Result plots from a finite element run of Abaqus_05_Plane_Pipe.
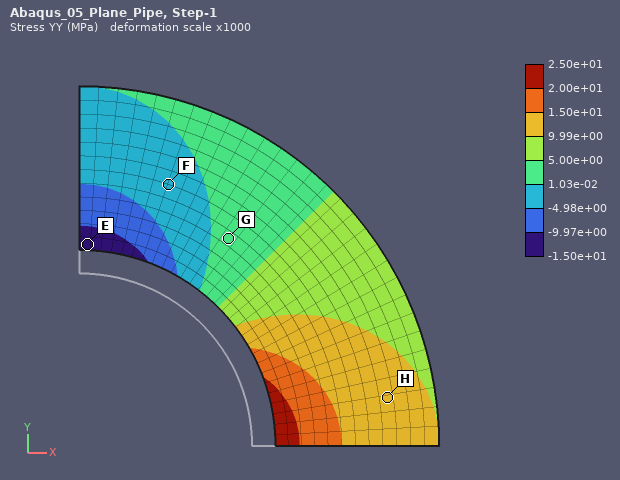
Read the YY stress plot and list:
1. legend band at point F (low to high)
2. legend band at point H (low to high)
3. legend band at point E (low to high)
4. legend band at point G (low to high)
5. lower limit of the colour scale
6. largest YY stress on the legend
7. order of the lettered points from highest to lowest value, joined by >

-4.98e+00 to 1.03e-02 MPa
9.99e+00 to 1.50e+01 MPa
-1.50e+01 to -9.97e+00 MPa
1.03e-02 to 5.00e+00 MPa
-1.50e+01 MPa
2.50e+01 MPa
H > G > F > E
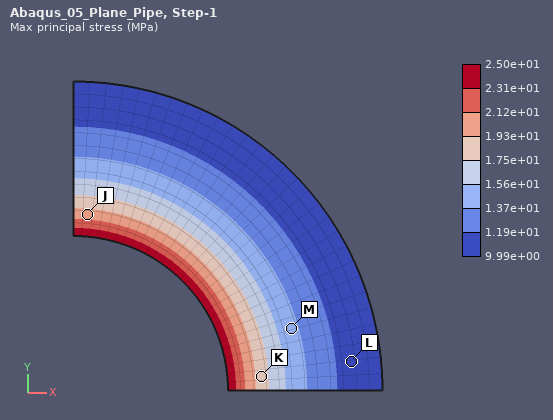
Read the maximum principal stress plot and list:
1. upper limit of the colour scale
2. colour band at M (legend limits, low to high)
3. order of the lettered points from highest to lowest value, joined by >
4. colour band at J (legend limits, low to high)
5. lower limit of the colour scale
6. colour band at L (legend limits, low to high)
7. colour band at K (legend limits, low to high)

2.50e+01 MPa
1.37e+01 to 1.56e+01 MPa
J > K > M > L
1.93e+01 to 2.12e+01 MPa
9.99e+00 MPa
9.99e+00 to 1.19e+01 MPa
1.75e+01 to 1.93e+01 MPa
